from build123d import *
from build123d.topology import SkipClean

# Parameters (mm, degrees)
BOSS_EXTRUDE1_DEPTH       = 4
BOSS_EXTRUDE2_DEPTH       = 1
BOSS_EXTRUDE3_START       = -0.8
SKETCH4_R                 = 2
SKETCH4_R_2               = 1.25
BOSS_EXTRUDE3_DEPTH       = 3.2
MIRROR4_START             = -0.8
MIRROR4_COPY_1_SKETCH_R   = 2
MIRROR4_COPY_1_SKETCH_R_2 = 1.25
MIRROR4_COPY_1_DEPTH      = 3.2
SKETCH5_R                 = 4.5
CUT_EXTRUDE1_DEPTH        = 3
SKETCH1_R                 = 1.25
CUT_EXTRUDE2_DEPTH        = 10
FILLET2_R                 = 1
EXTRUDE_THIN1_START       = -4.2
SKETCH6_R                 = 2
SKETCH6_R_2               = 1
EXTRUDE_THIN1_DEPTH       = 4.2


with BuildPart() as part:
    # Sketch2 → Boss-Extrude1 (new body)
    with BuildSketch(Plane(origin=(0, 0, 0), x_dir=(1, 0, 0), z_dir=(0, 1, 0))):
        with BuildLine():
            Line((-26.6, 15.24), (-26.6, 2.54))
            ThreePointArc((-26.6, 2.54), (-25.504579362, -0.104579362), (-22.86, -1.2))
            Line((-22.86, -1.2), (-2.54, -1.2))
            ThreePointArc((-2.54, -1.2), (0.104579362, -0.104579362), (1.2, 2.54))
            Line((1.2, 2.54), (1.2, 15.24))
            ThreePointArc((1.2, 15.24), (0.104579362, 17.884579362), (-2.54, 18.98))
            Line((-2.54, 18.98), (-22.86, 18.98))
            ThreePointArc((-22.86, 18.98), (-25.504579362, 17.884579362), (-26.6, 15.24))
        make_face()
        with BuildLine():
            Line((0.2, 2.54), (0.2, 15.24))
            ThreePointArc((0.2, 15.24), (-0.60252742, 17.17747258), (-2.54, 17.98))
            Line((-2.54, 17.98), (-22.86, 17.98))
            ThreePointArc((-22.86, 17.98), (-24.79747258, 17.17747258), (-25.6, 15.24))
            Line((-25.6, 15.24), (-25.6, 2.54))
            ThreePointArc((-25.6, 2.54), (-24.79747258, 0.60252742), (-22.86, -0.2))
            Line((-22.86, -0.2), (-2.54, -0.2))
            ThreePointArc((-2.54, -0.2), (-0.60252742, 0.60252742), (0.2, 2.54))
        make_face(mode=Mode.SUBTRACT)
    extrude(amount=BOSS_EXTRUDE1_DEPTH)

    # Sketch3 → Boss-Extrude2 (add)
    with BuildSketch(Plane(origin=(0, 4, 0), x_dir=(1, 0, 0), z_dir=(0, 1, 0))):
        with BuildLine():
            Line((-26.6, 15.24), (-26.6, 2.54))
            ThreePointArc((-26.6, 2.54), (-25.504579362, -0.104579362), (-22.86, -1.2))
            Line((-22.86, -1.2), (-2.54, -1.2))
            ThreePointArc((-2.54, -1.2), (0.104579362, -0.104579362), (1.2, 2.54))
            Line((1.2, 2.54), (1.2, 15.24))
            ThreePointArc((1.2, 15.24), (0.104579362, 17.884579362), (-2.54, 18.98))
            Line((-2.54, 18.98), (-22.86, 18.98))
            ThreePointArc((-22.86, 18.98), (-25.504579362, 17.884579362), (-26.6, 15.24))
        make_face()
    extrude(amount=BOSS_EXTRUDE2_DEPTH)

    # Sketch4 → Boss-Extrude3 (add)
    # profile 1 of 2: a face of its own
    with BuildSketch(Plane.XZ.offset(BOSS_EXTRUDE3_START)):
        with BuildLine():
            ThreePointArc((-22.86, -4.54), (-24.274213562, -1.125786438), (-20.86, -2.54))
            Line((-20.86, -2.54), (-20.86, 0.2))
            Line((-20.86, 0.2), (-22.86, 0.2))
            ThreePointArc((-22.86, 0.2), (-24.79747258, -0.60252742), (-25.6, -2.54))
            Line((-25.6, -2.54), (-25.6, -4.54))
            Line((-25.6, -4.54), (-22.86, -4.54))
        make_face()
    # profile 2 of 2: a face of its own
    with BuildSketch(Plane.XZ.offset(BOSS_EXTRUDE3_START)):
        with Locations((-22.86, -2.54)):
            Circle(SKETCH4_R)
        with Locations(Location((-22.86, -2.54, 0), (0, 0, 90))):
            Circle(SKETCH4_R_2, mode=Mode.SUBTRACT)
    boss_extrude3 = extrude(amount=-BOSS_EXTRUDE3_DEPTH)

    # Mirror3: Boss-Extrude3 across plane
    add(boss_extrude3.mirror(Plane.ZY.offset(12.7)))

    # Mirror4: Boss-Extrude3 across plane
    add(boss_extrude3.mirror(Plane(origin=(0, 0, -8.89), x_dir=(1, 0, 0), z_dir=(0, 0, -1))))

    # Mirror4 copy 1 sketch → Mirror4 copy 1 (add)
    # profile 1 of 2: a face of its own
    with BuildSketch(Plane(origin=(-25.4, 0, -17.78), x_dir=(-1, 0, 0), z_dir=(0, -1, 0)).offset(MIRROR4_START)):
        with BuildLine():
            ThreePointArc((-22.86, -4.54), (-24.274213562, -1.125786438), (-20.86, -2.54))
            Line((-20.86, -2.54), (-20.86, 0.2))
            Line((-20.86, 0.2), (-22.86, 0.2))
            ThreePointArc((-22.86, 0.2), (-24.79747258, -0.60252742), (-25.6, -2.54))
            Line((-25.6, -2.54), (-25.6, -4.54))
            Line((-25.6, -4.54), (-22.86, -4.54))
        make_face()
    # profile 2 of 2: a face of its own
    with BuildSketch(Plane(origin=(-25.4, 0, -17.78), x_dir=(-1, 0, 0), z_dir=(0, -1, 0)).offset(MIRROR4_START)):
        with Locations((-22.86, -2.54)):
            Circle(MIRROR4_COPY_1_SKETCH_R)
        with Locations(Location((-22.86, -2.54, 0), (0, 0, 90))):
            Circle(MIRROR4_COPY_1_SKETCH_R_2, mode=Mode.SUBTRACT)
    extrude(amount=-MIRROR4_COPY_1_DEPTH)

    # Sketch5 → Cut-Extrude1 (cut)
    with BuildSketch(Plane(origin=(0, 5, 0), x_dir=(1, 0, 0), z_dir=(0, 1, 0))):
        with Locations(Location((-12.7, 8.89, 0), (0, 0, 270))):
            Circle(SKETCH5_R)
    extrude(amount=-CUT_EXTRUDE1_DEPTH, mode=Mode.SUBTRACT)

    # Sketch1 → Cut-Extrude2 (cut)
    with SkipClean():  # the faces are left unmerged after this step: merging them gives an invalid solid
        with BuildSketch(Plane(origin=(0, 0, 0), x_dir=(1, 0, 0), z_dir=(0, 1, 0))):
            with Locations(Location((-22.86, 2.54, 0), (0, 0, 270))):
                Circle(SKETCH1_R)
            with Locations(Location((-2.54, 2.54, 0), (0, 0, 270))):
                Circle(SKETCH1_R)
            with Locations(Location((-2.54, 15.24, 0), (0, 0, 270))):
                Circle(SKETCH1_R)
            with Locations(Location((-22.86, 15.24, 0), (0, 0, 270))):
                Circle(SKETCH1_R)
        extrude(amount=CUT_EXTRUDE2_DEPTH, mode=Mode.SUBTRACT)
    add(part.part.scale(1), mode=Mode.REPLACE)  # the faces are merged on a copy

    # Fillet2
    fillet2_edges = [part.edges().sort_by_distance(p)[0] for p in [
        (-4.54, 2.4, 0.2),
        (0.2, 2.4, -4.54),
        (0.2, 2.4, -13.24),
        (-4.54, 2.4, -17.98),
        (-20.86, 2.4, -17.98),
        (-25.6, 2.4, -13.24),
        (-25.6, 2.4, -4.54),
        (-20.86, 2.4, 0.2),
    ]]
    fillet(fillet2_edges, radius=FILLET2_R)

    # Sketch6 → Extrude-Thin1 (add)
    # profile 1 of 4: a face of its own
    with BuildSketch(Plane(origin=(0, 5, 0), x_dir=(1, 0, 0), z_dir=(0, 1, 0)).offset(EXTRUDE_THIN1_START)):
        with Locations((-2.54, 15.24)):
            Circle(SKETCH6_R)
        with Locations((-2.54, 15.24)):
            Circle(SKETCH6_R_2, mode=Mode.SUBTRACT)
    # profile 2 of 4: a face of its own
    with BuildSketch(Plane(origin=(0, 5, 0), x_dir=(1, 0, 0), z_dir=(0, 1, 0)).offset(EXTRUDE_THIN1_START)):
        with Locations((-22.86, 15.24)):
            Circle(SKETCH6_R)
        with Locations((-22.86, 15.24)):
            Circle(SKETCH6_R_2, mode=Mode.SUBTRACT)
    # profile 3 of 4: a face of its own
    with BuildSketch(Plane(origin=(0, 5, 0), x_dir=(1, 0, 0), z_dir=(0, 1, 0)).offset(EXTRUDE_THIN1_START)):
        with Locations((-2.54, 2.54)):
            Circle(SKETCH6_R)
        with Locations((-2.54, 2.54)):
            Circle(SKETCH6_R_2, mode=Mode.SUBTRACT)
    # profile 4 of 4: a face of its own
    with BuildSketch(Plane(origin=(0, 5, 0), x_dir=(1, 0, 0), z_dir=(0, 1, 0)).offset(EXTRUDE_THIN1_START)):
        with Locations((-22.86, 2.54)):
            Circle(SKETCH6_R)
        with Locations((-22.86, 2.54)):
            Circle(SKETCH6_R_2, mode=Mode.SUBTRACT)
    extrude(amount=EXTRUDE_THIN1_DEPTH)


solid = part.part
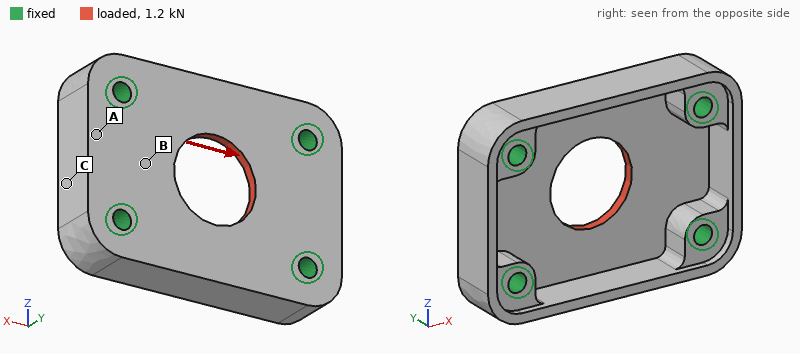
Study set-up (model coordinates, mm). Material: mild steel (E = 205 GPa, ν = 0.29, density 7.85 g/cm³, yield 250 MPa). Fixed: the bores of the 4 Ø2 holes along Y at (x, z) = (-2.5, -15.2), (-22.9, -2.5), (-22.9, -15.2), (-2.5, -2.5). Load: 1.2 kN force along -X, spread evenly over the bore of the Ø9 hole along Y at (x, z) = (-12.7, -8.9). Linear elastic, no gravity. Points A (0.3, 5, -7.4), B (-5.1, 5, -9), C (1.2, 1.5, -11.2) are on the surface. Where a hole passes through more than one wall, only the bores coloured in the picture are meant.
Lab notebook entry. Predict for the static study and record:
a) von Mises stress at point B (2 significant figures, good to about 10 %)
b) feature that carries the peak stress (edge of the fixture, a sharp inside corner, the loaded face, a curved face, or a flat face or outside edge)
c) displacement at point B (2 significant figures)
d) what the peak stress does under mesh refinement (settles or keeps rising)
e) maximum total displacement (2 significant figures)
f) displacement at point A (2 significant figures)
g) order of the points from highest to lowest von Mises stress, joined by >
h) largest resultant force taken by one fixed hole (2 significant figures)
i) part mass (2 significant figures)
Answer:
26 MPa
edge of the fixture
1.3 µm
keeps rising
1.8 µm
0.86 µm
B > A > C
310 N
8.2 g
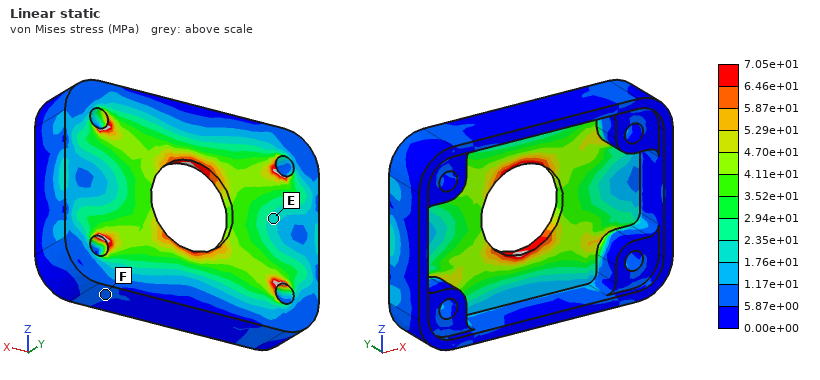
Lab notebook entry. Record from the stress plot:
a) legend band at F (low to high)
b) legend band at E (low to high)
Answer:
5.87e+00 to 1.17e+01 MPa
1.76e+01 to 2.35e+01 MPa
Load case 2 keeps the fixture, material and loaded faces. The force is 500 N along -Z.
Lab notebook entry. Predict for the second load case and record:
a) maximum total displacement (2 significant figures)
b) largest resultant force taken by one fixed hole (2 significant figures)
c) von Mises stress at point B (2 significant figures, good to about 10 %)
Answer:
1.8 µm
140 N
24 MPa
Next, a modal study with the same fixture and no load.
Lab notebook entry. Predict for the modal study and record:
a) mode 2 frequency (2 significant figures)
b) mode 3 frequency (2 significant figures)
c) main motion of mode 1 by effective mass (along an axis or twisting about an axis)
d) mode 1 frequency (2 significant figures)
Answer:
30 kHz
35 kHz
along Y
23 kHz
